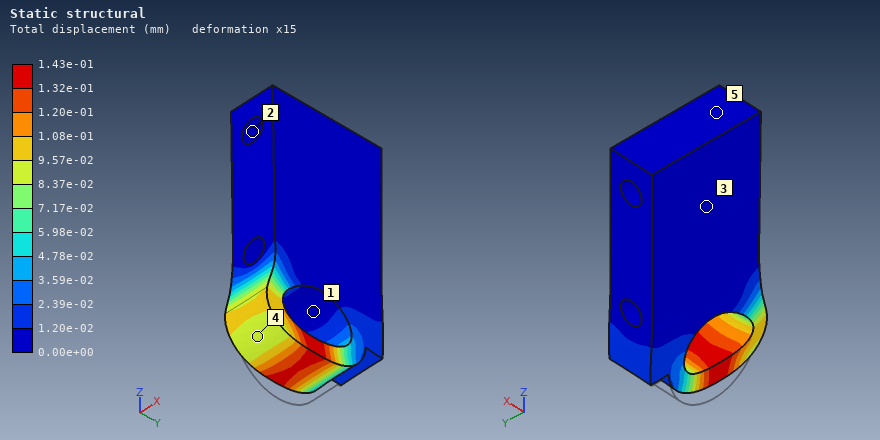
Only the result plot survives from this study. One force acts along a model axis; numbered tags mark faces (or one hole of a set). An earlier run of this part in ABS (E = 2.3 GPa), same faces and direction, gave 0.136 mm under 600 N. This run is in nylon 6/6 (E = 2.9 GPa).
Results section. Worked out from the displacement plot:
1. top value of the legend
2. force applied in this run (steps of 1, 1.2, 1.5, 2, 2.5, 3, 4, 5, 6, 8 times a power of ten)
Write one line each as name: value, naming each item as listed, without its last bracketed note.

top value of the legend: 1.43e-01 mm
force applied in this run: 800 N
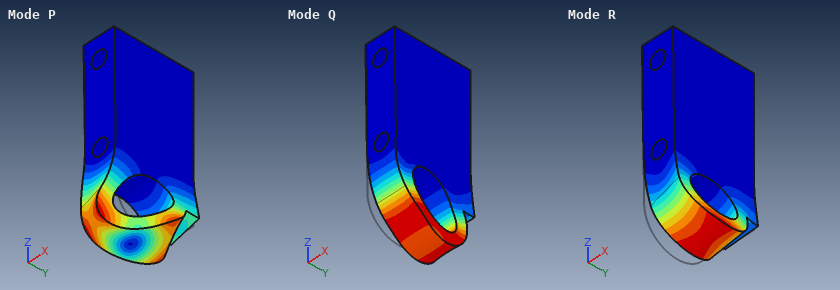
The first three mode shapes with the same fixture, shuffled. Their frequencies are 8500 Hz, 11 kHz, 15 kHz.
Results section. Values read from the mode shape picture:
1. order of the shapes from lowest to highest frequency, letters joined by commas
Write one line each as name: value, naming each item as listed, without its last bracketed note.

order of the shapes from lowest to highest frequency, letters joined by commas: R, Q, P
